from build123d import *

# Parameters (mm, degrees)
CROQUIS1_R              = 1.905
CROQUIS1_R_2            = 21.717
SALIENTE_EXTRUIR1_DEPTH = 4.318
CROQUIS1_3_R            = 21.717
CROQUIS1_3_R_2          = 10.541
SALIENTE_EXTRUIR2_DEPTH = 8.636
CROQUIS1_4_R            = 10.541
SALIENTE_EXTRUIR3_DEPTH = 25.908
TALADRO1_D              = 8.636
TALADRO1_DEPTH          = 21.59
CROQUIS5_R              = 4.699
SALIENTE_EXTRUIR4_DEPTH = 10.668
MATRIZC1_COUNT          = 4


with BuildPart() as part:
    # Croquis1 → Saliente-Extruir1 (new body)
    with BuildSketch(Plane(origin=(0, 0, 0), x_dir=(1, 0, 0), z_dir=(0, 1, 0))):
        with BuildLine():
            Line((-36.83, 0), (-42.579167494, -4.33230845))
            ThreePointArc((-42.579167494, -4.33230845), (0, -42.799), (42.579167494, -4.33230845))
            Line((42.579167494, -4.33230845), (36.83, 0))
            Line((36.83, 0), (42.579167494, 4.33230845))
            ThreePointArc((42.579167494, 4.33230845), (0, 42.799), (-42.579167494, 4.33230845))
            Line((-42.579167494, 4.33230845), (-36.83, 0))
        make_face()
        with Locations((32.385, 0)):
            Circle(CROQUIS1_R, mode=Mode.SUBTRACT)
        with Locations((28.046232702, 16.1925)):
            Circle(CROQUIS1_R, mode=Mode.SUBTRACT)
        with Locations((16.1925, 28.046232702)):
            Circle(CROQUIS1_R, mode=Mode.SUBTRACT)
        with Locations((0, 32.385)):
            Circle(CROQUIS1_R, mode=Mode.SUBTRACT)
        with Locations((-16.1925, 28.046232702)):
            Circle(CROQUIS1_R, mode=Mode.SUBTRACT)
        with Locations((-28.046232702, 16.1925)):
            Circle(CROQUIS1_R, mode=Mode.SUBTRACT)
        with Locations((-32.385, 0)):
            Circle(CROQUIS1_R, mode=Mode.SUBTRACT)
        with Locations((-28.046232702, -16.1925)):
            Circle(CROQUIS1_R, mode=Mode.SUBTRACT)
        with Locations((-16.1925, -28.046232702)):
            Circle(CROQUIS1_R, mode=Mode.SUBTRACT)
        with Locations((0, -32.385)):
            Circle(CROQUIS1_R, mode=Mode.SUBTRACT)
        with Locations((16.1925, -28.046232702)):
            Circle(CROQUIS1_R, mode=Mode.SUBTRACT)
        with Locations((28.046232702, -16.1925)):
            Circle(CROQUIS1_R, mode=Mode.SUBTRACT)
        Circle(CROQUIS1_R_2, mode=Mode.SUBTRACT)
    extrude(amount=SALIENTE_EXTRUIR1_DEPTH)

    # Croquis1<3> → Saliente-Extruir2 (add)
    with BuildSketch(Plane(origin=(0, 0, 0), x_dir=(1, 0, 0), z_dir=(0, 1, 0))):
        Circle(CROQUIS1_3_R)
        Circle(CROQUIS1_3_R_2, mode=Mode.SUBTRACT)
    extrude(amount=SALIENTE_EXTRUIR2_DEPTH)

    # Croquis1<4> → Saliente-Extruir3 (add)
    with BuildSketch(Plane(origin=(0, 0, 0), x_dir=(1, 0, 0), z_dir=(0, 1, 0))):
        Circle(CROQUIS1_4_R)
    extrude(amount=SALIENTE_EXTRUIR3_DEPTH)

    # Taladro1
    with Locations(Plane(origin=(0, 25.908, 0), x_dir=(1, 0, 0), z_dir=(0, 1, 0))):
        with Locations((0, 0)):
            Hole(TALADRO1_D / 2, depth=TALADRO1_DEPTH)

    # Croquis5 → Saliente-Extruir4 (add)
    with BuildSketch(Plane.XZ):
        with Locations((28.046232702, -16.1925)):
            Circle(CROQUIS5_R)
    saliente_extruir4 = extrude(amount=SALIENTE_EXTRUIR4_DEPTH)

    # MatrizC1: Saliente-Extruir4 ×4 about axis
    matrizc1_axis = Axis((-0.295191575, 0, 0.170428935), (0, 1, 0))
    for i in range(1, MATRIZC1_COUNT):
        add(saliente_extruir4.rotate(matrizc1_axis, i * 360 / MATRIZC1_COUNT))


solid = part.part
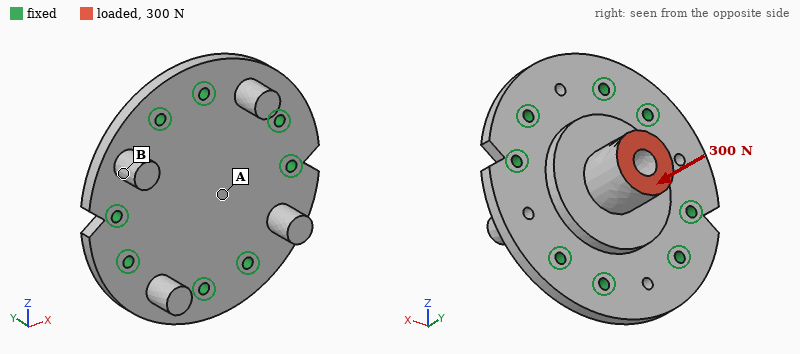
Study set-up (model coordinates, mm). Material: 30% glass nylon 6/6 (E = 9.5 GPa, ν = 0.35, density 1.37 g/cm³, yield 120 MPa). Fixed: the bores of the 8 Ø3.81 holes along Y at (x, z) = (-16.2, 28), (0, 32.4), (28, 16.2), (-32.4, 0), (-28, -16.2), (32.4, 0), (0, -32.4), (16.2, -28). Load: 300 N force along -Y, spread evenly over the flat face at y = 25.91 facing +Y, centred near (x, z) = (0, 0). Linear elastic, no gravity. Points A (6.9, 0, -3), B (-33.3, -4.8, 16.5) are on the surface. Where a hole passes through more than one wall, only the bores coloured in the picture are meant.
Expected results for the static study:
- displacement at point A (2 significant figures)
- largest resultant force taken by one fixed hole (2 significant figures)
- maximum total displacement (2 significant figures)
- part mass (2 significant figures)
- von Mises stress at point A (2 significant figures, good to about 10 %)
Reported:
16 µm
52 N
17 µm
52 g
1.9 MPa
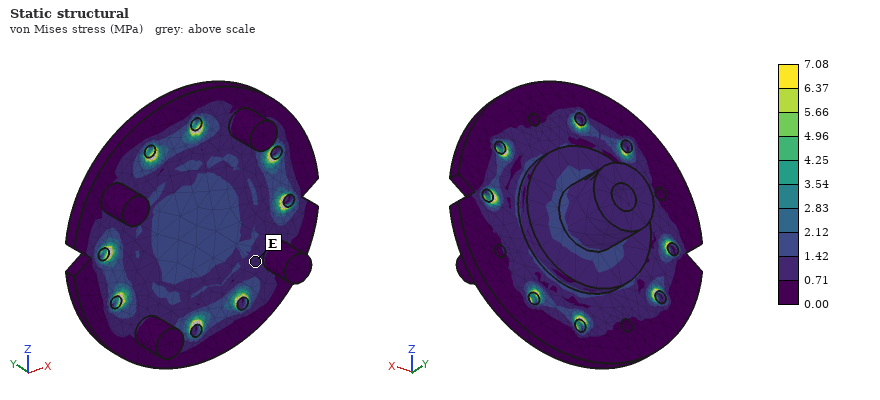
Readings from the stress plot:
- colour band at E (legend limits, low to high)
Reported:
0.71 to 1.42 MPa
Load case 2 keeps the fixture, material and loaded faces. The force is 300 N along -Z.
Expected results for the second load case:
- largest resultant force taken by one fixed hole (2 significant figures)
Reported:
95 N
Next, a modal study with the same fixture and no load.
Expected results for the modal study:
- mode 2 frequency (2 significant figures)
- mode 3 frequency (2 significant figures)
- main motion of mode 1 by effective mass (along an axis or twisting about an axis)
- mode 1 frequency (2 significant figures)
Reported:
5700 Hz
5900 Hz
along Y
4700 Hz
